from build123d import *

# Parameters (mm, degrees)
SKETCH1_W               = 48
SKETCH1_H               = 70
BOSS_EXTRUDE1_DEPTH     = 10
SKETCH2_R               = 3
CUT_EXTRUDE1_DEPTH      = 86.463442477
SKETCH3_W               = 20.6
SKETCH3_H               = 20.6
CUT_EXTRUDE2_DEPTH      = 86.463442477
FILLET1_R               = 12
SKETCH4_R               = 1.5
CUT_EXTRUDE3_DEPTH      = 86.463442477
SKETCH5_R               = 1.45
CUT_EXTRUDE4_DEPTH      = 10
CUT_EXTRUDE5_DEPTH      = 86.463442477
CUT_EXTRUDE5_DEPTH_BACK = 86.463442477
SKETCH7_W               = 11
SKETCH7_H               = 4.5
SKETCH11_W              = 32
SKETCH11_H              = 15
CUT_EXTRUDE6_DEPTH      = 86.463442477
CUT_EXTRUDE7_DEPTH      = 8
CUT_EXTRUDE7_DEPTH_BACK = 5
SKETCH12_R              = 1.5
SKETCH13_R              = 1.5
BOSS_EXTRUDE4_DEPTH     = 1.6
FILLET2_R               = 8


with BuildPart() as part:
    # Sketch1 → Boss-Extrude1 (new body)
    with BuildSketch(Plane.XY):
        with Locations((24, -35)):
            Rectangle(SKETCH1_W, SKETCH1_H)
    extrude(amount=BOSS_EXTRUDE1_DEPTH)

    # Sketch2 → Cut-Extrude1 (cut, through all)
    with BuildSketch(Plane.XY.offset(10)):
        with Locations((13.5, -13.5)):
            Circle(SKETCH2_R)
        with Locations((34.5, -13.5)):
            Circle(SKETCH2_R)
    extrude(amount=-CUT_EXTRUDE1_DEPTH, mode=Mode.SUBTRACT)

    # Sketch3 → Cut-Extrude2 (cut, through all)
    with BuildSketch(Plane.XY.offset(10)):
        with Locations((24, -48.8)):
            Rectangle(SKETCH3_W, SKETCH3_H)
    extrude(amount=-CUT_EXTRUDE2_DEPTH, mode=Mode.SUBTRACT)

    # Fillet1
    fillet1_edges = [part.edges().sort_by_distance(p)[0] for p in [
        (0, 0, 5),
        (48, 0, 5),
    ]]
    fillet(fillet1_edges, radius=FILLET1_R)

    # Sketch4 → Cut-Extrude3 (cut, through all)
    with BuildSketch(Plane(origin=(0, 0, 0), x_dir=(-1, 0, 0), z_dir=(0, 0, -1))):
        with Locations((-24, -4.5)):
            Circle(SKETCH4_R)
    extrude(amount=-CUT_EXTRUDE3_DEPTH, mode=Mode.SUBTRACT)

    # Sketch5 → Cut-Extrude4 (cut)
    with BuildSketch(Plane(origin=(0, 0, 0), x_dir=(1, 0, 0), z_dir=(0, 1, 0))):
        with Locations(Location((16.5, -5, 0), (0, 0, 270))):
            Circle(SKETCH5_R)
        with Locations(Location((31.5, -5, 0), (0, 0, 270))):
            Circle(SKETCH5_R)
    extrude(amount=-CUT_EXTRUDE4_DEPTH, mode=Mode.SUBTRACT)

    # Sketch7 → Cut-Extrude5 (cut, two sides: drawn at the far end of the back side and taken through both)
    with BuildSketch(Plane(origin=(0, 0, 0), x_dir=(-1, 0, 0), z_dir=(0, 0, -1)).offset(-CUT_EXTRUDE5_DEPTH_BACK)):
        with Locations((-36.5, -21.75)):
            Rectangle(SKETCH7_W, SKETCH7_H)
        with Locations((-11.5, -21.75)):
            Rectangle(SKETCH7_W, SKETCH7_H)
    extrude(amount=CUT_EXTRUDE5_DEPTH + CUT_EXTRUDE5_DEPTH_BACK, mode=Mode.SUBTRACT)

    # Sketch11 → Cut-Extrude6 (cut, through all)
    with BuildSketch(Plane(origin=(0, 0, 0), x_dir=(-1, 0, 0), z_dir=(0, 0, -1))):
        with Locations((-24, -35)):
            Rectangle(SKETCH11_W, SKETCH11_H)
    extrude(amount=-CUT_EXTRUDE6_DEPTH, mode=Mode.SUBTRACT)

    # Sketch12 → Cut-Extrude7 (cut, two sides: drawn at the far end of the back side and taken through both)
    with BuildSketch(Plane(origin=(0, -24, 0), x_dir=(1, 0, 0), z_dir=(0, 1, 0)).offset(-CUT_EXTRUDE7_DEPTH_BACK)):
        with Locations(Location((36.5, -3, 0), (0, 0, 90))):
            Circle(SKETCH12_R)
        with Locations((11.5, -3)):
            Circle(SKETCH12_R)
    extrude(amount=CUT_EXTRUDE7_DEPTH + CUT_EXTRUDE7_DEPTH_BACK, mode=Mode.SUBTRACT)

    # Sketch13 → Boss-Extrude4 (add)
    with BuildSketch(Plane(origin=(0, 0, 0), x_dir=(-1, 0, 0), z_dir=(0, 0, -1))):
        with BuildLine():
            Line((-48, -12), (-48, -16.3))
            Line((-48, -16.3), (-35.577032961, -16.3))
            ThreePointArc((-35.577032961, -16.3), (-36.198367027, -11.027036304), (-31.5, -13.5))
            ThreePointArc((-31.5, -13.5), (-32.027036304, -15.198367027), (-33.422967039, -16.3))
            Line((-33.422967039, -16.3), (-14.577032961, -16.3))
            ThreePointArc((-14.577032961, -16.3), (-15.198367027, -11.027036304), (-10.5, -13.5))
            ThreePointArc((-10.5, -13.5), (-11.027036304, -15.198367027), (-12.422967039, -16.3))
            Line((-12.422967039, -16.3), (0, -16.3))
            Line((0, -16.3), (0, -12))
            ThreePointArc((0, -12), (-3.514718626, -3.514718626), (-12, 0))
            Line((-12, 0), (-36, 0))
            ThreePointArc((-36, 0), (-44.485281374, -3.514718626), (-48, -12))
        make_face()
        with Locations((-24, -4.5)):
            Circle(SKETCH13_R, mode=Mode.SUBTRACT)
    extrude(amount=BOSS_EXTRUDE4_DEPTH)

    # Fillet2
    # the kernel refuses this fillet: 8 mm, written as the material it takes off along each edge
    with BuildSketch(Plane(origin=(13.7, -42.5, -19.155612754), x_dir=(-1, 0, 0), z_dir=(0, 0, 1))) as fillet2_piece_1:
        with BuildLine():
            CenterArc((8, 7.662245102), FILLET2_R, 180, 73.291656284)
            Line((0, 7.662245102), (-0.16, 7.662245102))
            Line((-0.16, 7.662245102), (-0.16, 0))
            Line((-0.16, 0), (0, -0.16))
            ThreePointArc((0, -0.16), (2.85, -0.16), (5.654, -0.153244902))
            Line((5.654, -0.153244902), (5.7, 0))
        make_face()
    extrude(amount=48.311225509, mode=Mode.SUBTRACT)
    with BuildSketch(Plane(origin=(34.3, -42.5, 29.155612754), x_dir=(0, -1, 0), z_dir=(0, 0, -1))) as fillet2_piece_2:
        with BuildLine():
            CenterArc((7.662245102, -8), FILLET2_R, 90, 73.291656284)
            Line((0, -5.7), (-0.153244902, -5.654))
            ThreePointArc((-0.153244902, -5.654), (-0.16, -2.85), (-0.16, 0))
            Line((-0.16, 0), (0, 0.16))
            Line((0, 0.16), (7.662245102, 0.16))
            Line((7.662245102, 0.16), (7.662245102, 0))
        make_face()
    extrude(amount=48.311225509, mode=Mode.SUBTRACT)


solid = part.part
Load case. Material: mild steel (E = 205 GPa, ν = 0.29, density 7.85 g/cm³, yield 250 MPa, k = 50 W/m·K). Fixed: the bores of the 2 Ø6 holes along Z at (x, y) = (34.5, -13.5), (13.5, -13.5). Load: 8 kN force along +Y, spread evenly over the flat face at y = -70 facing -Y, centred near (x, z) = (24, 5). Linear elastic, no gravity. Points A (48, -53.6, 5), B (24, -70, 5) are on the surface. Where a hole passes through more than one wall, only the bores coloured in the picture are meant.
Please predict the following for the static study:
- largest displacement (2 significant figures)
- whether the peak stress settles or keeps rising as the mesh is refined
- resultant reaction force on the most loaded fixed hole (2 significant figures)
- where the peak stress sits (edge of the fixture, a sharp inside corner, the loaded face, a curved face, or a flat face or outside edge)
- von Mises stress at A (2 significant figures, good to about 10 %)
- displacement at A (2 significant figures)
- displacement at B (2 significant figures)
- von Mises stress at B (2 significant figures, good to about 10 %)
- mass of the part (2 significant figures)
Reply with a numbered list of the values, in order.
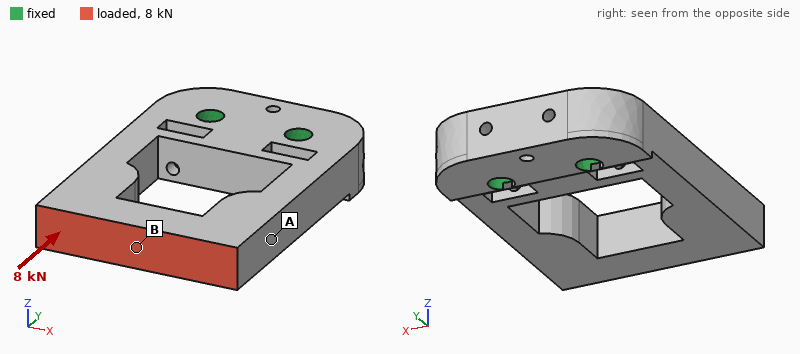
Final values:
1. 23 µm
2. keeps rising
3. 4.1 kN
4. edge of the fixture
5. 20 MPa
6. 13 µm
7. 23 µm
8. 57 MPa
9. 190 g
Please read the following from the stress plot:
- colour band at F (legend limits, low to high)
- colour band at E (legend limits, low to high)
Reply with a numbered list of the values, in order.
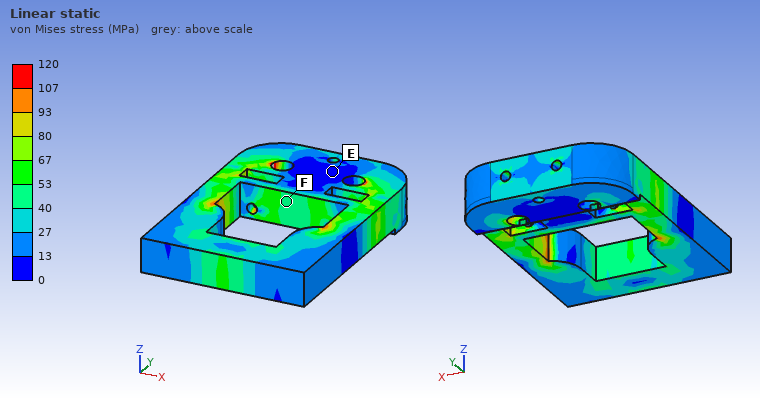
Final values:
1. 40 to 53 MPa
2. 0 to 13 MPa
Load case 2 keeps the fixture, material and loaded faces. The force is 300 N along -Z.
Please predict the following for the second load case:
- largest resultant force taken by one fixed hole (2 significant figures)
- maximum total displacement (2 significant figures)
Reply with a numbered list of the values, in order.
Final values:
1. 150 N
2. 70 µm
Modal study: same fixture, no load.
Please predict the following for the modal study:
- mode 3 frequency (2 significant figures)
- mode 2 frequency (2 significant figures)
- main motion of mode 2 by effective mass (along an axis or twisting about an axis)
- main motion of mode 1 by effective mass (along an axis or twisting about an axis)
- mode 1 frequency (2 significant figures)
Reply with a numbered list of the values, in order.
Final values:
1. 3900 Hz
2. 3700 Hz
3. along X
4. along Z
5. 1600 Hz
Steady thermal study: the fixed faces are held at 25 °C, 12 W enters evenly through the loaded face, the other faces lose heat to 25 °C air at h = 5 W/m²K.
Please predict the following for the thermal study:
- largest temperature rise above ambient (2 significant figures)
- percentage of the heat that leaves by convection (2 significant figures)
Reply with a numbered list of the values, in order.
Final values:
1. 64 K
2. 8.9 %
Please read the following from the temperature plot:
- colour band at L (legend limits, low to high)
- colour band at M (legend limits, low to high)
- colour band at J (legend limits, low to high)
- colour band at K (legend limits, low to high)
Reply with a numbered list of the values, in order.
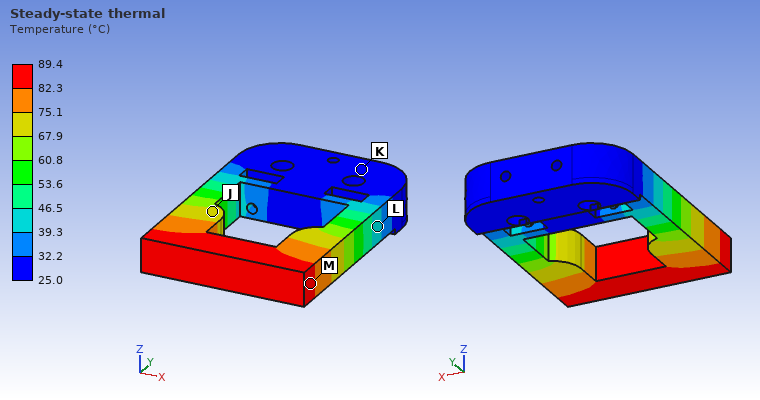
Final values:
1. 39.3 to 46.5 °C
2. 82.3 to 89.4 °C
3. 67.9 to 75.1 °C
4. 25.0 to 32.2 °C
